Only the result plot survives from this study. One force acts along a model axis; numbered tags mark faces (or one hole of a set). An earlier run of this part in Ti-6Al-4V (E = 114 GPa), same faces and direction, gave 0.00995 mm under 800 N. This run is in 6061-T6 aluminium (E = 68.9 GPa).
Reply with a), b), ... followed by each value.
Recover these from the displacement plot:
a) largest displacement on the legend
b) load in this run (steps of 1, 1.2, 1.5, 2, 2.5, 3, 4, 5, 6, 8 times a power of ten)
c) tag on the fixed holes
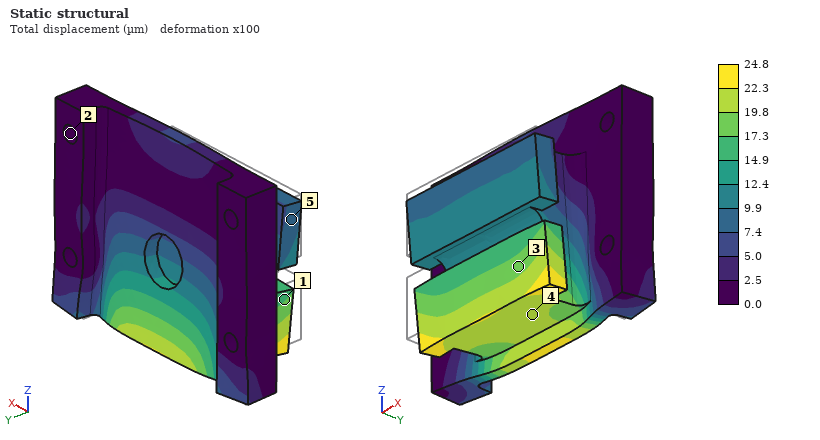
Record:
a) 24.8 µm
b) 1.2 kN
c) 2
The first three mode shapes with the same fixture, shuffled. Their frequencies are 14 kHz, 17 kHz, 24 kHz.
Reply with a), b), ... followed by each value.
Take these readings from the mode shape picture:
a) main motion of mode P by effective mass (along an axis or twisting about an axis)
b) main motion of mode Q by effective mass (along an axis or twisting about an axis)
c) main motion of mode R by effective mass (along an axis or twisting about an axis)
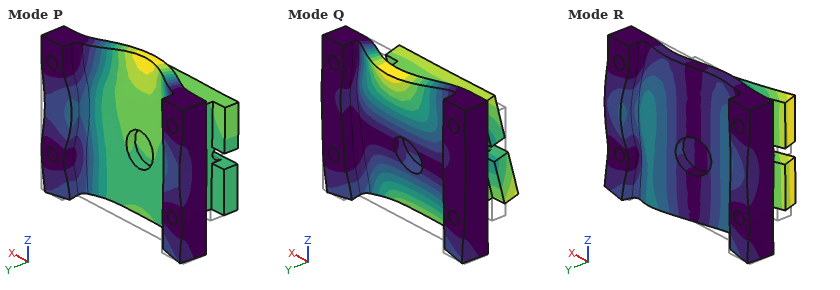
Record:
a) along Y
b) along Z
c) along X
